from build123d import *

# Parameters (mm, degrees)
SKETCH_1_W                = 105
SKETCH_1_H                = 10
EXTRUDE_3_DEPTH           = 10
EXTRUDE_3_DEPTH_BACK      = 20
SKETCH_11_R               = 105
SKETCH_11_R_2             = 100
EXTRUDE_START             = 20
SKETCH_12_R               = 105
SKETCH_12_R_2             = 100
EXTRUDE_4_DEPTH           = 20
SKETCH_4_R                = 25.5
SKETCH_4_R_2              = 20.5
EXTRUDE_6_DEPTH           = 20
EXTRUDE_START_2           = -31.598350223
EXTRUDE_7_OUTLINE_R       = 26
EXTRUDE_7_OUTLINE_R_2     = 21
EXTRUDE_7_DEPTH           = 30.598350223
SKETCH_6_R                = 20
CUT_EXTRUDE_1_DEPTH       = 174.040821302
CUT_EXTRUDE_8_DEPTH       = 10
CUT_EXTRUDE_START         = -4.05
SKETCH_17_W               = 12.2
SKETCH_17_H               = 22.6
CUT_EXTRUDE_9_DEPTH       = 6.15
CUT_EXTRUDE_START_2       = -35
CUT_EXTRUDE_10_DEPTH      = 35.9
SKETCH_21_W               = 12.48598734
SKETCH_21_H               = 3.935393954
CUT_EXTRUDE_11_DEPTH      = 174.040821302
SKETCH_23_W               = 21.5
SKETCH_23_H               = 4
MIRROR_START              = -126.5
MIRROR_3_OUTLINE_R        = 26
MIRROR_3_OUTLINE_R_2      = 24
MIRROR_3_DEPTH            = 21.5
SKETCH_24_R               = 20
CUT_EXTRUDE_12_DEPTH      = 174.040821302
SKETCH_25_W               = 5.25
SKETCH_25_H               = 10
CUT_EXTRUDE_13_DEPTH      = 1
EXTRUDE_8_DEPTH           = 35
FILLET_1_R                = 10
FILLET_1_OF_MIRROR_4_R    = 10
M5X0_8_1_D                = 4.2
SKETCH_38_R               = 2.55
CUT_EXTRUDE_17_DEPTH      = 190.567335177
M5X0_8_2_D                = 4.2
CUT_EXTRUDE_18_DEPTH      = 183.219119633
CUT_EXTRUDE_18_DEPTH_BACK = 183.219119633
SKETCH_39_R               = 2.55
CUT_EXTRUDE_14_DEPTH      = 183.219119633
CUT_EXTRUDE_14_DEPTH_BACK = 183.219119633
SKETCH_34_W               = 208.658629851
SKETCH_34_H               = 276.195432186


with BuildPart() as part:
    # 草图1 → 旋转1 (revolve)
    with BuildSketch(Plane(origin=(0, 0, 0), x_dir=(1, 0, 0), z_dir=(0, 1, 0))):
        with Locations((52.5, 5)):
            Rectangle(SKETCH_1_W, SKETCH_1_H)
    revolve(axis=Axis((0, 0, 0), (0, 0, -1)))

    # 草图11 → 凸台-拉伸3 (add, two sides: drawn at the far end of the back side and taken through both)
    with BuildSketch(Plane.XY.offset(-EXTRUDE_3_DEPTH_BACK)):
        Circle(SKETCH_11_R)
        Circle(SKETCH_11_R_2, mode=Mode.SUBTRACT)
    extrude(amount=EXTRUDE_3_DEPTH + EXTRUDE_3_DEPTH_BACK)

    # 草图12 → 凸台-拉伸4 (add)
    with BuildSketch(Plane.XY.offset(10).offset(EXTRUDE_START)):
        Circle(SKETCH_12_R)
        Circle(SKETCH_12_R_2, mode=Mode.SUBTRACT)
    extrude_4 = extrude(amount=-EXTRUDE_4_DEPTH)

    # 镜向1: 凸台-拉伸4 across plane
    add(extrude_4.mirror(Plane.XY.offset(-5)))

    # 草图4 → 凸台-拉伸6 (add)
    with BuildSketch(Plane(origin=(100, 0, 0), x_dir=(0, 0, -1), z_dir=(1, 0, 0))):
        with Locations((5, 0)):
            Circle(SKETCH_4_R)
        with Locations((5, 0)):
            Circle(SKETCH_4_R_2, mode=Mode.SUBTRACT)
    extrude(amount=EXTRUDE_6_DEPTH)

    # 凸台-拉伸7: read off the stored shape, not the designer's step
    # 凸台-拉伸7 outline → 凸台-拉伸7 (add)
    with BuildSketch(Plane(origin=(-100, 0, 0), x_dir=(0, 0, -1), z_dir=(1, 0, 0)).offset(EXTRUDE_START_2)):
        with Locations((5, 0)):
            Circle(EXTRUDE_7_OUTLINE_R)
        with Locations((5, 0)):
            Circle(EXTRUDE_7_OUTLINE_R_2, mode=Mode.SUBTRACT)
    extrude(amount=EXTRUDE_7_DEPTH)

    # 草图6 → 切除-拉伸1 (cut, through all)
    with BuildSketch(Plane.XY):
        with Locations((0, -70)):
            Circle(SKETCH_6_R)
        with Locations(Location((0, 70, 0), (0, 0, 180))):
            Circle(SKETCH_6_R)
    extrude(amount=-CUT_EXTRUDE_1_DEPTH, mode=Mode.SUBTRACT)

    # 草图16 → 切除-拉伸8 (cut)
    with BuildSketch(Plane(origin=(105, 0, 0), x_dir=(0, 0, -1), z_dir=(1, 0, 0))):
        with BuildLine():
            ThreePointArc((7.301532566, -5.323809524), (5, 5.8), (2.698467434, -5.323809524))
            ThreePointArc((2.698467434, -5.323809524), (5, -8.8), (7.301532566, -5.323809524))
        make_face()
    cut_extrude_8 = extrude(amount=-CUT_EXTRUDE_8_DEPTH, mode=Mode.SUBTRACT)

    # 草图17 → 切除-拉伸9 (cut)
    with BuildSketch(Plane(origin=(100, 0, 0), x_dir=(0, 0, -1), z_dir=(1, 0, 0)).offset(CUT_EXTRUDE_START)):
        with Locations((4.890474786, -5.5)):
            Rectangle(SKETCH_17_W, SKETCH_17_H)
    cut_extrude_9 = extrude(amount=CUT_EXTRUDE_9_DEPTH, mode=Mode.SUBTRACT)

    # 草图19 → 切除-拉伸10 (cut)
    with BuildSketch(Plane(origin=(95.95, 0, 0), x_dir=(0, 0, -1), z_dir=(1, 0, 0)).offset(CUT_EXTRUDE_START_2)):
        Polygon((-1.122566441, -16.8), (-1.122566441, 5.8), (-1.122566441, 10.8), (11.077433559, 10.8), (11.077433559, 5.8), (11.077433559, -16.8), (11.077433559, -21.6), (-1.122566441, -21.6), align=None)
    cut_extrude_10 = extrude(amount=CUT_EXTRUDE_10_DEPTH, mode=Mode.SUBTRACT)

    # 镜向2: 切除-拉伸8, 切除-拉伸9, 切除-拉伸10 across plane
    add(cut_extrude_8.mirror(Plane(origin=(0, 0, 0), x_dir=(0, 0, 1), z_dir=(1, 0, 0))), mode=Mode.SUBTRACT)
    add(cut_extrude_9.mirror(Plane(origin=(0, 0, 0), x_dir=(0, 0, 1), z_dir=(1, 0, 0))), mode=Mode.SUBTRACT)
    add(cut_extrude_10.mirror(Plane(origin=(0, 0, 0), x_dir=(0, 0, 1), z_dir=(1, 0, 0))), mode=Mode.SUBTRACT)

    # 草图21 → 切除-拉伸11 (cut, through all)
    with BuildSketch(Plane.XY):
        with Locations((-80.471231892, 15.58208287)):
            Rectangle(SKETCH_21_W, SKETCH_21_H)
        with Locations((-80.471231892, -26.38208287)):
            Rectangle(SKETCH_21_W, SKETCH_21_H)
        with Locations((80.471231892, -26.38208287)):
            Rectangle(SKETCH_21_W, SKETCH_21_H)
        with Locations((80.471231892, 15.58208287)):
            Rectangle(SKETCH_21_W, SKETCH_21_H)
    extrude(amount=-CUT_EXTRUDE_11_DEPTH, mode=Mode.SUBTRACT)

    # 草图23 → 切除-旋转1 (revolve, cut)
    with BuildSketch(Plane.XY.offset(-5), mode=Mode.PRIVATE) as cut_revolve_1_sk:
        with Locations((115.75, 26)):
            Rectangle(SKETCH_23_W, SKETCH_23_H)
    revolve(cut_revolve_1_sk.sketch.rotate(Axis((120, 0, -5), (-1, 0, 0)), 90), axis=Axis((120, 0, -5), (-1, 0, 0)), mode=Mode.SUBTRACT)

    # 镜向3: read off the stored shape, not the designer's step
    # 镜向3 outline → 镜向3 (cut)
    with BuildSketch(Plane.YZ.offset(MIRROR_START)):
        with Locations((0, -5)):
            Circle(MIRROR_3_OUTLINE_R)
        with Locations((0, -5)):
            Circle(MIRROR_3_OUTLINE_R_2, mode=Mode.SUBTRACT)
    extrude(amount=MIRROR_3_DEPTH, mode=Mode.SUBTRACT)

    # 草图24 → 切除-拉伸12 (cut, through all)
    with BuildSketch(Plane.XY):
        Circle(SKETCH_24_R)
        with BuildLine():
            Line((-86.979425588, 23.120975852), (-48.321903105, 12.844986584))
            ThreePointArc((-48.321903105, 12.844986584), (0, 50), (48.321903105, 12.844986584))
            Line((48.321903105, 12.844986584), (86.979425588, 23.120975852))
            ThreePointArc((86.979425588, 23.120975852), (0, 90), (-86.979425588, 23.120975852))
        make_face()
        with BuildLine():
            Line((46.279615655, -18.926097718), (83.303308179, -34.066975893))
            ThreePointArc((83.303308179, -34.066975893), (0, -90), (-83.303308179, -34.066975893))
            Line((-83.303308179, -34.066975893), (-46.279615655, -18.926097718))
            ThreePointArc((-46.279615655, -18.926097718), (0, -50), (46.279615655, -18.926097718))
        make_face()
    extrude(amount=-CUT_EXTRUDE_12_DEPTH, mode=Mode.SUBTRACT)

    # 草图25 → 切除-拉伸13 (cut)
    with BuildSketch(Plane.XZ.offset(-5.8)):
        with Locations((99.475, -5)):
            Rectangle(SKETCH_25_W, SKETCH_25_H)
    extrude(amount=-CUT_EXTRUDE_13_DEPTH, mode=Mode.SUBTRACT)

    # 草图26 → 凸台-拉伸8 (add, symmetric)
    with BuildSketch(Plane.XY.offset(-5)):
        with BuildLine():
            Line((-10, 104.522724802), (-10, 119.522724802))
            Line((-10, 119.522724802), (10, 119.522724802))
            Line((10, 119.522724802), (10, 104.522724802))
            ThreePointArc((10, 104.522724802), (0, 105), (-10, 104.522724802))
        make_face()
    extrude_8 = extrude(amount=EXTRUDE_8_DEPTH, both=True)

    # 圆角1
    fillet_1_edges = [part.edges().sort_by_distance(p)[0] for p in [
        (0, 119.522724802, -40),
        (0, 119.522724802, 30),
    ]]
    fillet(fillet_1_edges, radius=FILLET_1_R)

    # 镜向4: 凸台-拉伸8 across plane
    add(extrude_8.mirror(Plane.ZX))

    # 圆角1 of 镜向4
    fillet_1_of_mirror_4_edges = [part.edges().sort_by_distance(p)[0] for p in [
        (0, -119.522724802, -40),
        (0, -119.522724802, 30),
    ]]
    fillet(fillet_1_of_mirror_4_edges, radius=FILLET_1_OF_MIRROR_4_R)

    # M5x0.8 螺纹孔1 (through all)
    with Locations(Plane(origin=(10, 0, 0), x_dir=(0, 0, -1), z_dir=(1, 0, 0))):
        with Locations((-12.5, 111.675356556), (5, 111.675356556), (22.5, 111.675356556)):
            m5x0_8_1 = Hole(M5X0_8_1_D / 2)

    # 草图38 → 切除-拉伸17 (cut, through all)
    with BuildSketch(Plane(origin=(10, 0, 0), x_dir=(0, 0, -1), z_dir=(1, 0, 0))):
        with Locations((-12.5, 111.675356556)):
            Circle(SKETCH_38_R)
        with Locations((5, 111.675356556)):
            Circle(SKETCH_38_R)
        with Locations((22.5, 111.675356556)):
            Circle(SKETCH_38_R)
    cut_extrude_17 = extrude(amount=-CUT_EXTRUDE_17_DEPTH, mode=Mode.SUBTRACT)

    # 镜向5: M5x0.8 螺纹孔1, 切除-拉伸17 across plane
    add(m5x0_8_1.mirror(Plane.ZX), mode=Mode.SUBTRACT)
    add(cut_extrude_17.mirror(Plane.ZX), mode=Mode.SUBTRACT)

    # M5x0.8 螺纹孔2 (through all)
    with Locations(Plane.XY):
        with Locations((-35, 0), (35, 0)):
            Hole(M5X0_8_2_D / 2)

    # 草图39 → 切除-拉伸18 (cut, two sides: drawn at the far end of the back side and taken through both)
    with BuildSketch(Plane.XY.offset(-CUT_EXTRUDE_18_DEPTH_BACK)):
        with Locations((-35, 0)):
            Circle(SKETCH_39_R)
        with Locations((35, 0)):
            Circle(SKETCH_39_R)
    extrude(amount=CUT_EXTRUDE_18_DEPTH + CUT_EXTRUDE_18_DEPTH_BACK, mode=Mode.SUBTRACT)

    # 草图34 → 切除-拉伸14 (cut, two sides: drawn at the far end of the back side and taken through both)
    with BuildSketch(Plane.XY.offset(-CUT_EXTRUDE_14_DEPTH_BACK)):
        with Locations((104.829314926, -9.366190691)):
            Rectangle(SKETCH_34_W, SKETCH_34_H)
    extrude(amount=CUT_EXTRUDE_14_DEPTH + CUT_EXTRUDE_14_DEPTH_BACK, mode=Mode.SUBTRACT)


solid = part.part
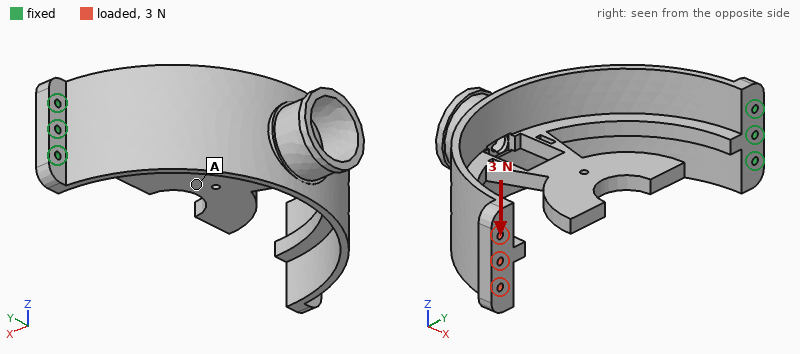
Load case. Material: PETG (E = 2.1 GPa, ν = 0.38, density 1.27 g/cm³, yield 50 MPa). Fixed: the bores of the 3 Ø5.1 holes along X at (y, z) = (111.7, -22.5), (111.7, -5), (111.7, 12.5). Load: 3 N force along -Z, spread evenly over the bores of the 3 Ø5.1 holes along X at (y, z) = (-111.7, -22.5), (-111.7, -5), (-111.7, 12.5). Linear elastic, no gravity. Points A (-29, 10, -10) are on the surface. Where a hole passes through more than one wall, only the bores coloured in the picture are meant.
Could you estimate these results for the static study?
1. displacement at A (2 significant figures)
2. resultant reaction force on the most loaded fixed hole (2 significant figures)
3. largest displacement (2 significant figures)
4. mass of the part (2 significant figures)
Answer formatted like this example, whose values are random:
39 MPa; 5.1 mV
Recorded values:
1.0 mm; 18 N; 2.7 mm; 270 g
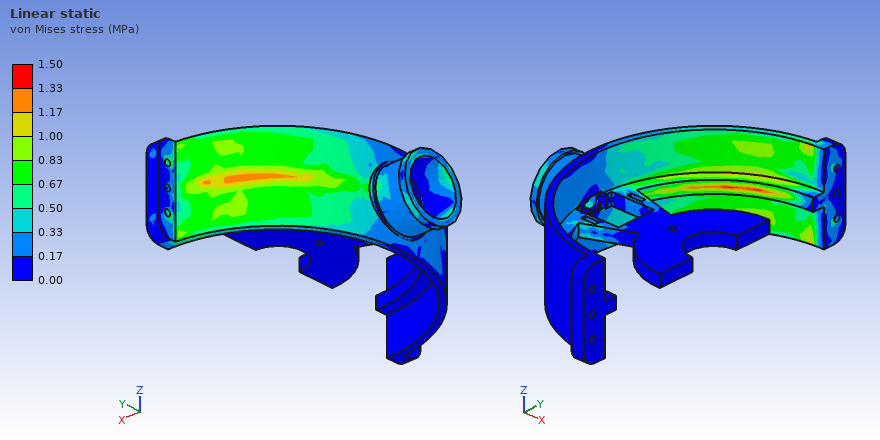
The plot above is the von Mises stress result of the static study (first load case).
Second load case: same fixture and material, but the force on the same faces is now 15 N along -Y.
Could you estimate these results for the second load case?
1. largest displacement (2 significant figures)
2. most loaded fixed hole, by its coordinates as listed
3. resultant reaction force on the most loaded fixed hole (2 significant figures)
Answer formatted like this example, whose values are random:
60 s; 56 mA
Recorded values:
3.4 mm; (111.7, -5); 12 N
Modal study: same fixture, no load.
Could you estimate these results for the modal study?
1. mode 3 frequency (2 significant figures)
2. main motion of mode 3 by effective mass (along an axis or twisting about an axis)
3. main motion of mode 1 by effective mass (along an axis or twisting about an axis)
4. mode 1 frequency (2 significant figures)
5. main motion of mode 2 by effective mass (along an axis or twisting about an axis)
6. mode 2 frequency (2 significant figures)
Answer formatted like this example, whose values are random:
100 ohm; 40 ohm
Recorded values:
69 Hz; along Y; along Z; 22 Hz; along X; 24 Hz
